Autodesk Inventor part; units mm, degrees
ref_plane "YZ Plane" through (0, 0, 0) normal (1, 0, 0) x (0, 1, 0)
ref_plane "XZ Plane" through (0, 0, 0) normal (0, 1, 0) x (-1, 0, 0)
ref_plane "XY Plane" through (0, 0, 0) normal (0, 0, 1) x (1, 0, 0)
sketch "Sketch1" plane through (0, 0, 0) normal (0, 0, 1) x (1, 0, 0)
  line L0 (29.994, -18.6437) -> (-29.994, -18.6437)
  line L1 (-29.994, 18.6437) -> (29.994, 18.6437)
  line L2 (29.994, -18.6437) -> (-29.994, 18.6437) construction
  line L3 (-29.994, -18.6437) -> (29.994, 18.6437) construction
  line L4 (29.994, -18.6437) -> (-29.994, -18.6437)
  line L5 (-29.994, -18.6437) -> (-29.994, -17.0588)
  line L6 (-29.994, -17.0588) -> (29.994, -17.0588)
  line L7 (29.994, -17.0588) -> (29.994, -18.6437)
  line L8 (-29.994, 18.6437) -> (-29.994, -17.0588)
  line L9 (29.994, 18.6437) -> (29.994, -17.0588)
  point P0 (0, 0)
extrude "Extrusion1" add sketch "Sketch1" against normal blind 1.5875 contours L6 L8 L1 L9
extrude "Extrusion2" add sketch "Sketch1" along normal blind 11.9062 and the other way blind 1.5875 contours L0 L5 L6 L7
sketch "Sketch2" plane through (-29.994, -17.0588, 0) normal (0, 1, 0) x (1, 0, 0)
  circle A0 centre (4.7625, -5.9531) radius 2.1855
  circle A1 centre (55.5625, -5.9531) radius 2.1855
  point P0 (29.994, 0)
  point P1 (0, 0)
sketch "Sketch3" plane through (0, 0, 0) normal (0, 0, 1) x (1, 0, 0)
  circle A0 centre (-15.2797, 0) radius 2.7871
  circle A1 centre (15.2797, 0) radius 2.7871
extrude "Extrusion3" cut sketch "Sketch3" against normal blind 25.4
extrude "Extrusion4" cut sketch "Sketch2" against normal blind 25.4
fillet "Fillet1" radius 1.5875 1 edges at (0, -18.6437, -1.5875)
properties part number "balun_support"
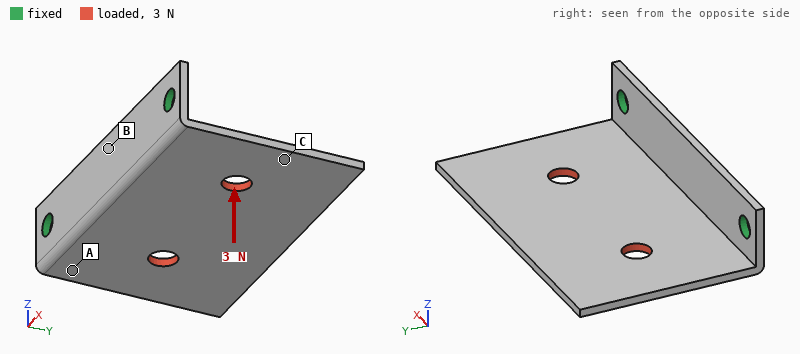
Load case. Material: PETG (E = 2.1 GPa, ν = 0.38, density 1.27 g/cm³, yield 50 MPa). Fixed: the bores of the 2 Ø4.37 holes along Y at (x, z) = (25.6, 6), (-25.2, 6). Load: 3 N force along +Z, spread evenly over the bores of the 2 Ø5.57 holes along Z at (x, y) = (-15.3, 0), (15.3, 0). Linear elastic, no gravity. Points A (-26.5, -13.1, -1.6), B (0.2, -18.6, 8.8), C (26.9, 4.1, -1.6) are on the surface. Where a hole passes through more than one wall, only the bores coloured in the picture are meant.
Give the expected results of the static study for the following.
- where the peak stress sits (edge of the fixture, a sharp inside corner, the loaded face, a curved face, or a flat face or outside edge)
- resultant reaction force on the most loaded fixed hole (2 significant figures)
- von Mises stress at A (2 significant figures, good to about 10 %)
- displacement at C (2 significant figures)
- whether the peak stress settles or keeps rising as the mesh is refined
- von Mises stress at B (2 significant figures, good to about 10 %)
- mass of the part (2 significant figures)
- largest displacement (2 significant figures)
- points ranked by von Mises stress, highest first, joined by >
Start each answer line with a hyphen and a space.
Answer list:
- edge of the fixture
- 1.6 N
- 1.8 MPa
- 0.39 mm
- keeps rising
- 0.71 MPa
- 5.7 g
- 0.74 mm
- A > B > C
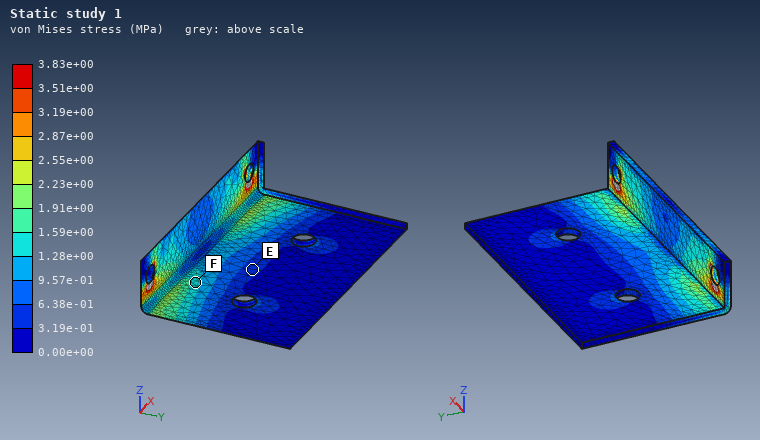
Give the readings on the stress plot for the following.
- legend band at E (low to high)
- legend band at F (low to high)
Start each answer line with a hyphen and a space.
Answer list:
- 3.19e-01 to 6.38e-01 MPa
- 1.28e+00 to 1.59e+00 MPa
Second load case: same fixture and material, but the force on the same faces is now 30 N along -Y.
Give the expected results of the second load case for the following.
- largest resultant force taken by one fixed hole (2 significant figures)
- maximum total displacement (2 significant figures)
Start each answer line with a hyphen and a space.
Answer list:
- 15 N
- 0.65 mm
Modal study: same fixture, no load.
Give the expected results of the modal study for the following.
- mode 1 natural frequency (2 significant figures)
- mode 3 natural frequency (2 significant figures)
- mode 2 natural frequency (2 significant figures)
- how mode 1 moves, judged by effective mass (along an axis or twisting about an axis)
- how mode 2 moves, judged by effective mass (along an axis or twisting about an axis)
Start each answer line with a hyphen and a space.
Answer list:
- 180 Hz
- 860 Hz
- 380 Hz
- along Z
- twisting about Y
